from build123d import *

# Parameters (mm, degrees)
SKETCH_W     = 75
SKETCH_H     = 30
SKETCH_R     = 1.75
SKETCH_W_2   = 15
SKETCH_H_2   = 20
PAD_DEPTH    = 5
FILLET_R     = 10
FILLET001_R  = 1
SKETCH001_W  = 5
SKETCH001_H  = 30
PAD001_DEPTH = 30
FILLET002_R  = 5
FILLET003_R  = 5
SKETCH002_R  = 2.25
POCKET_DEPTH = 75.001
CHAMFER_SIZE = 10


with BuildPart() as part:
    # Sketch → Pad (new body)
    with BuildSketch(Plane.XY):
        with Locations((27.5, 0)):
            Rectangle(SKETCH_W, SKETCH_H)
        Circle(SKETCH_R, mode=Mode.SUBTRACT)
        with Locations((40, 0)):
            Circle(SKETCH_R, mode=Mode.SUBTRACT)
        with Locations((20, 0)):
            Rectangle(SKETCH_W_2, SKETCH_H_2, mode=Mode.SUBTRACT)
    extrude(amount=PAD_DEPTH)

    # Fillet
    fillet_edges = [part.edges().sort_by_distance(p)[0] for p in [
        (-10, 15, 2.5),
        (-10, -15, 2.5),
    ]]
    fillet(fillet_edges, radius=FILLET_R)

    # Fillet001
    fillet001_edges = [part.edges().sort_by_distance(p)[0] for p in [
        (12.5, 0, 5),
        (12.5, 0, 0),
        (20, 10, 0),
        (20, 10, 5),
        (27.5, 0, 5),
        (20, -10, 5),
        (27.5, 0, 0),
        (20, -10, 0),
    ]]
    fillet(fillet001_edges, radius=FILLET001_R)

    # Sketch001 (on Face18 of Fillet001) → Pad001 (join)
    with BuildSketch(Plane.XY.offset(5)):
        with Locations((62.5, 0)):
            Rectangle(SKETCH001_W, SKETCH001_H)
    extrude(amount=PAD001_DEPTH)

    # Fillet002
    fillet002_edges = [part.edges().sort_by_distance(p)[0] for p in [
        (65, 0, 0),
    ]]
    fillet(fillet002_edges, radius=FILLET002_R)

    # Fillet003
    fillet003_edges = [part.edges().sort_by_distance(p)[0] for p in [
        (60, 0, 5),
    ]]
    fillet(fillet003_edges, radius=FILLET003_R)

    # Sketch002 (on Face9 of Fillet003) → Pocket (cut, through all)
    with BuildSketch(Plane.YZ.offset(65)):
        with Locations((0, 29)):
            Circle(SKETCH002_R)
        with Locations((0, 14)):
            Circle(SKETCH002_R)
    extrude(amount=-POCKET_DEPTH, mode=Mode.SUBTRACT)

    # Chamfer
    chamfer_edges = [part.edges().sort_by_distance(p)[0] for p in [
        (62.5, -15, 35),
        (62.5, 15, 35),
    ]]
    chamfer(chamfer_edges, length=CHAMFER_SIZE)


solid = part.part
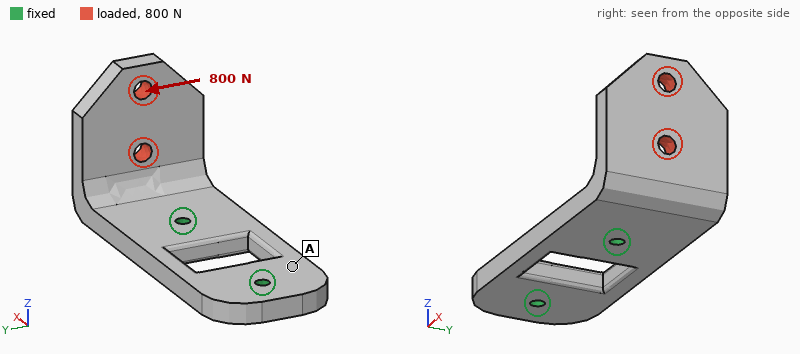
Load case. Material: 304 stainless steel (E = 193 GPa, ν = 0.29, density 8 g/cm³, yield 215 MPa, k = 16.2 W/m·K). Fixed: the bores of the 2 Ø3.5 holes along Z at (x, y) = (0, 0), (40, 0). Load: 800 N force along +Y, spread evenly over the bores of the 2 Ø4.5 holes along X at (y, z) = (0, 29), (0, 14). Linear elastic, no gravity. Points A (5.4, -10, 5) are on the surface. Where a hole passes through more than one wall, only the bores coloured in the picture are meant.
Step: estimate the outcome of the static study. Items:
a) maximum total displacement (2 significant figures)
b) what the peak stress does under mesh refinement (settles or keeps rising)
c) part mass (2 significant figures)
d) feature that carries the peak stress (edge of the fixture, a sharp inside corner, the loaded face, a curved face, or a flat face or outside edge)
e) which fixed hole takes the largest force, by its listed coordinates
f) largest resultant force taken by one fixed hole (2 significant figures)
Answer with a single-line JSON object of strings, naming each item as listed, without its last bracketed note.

{"maximum total displacement": "0.13 mm", "what the peak stress does under mesh refinement": "keeps rising", "part mass": "110 g", "feature that carries the peak stress": "edge of the fixture", "which fixed hole takes the largest force, by its listed coordinates": "(40, 0)", "largest resultant force taken by one fixed hole": "1.0 kN"}
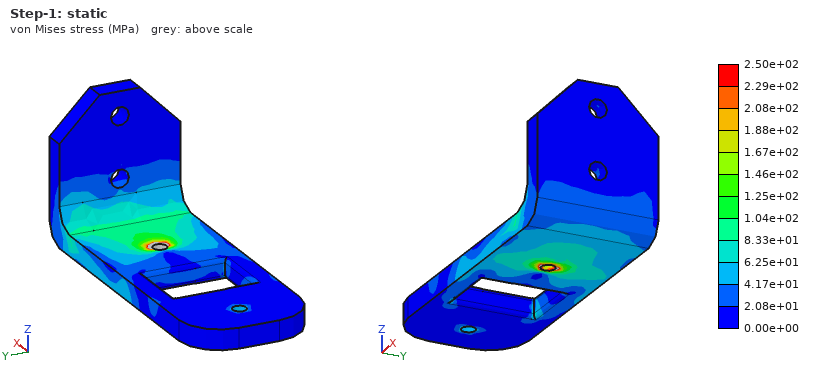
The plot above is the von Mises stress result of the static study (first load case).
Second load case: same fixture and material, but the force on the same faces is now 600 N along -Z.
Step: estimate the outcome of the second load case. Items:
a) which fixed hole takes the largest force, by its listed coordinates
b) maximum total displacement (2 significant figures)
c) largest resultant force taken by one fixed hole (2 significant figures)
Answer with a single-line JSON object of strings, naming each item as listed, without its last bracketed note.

{"which fixed hole takes the largest force, by its listed coordinates": "(40, 0)", "maximum total displacement": "0.11 mm", "largest resultant force taken by one fixed hole": "680 N"}
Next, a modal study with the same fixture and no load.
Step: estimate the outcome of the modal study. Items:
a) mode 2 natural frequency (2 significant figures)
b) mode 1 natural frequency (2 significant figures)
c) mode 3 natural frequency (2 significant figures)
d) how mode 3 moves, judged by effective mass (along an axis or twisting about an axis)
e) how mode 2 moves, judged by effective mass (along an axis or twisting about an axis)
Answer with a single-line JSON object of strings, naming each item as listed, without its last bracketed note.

{"mode 2 natural frequency": "2800 Hz", "mode 1 natural frequency": "1900 Hz", "mode 3 natural frequency": "5700 Hz", "how mode 3 moves, judged by effective mass": "along Z", "how mode 2 moves, judged by effective mass": "along Y"}
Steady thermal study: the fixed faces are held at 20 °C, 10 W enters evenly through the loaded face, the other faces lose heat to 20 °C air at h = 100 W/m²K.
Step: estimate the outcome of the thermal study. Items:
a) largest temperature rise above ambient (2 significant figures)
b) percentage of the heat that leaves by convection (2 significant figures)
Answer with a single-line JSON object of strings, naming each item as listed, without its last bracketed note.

{"largest temperature rise above ambient": "58 K", "percentage of the heat that leaves by convection": "87 %"}
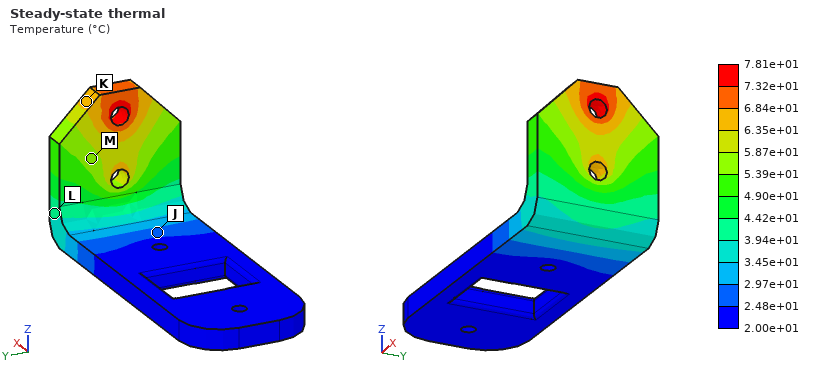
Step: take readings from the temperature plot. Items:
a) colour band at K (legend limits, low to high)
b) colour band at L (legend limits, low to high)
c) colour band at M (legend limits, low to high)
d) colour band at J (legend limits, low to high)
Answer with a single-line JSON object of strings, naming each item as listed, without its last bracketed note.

{"colour band at K": "6.35e+01 to 6.84e+01 °C", "colour band at L": "3.94e+01 to 4.42e+01 °C", "colour band at M": "5.39e+01 to 5.87e+01 °C", "colour band at J": "2.48e+01 to 2.97e+01 °C"}
